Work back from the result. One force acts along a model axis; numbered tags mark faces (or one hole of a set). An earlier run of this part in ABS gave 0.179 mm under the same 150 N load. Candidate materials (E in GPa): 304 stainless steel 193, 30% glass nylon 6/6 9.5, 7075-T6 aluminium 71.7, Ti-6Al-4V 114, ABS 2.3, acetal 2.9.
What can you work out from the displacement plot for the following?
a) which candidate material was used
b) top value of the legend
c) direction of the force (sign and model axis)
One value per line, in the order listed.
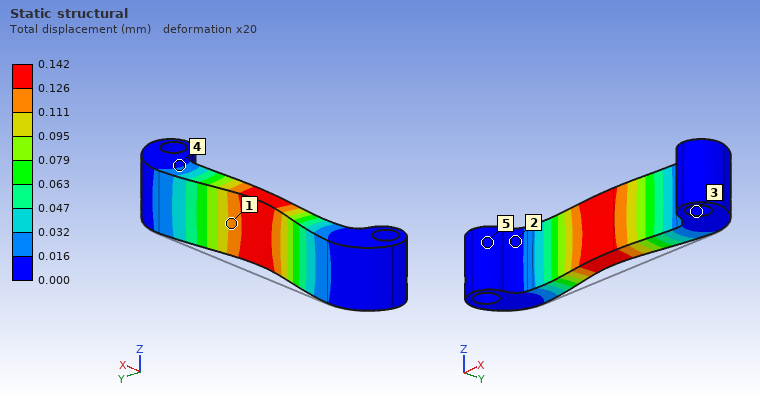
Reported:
acetal
0.142 mm
-Y
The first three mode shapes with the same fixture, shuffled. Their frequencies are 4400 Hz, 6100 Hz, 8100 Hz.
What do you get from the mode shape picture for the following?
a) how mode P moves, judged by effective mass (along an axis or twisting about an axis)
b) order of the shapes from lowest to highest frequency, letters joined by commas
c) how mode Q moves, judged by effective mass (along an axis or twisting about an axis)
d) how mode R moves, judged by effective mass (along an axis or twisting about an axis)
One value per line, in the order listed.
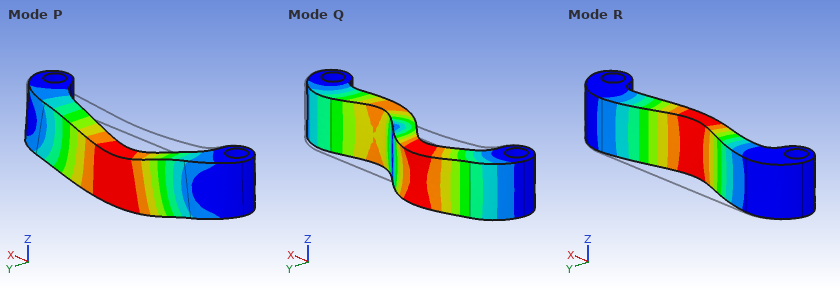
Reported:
along Z
R, P, Q
along X
along Y
